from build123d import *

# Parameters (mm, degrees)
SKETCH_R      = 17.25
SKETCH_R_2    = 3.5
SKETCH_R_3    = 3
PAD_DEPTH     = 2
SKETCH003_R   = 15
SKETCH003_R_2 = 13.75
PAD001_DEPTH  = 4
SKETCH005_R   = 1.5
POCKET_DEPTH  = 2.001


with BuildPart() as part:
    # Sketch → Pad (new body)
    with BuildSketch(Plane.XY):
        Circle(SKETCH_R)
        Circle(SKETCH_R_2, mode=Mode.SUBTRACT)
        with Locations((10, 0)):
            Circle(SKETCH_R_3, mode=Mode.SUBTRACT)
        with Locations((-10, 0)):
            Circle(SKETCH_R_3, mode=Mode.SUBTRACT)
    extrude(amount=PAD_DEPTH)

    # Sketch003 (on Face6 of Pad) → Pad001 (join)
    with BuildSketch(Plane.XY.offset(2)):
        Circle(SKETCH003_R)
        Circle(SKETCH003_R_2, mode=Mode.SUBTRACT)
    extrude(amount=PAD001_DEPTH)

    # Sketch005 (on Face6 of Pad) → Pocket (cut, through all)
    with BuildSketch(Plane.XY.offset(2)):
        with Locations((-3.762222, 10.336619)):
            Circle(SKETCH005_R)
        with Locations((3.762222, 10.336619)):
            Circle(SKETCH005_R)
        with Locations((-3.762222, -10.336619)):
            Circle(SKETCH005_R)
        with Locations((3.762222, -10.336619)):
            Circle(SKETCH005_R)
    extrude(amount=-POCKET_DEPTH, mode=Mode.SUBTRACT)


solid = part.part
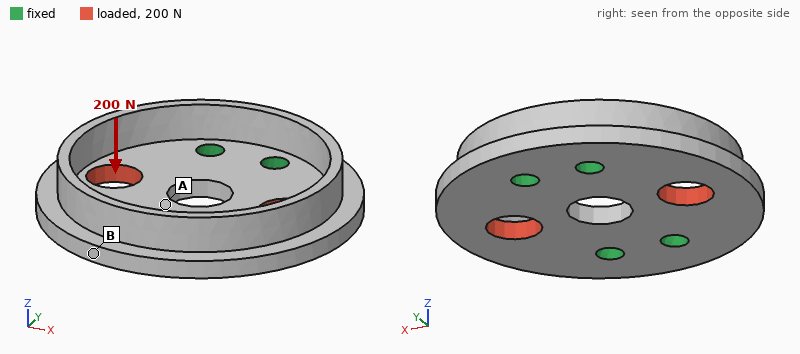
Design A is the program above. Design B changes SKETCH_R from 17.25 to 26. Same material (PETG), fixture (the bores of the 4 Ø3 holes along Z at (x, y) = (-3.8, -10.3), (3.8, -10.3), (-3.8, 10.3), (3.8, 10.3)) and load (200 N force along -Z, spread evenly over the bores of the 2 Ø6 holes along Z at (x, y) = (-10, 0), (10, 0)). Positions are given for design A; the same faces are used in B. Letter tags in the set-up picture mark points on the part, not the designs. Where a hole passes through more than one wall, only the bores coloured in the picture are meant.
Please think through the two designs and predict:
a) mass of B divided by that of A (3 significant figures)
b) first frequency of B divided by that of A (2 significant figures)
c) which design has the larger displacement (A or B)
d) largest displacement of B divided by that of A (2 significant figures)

2.15
0.40
B
1.2
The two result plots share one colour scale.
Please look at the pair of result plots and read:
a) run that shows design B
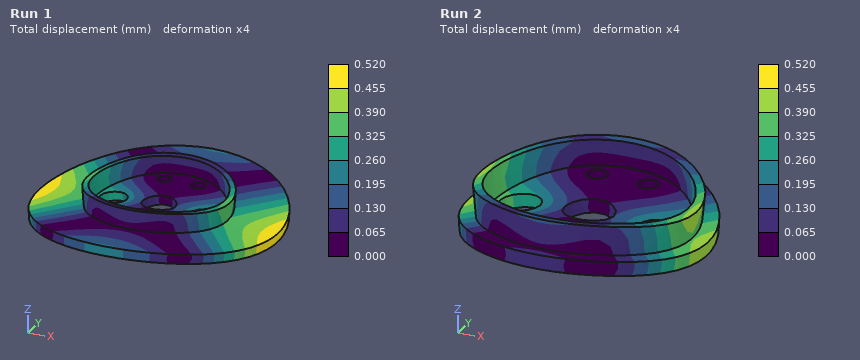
Run 1
